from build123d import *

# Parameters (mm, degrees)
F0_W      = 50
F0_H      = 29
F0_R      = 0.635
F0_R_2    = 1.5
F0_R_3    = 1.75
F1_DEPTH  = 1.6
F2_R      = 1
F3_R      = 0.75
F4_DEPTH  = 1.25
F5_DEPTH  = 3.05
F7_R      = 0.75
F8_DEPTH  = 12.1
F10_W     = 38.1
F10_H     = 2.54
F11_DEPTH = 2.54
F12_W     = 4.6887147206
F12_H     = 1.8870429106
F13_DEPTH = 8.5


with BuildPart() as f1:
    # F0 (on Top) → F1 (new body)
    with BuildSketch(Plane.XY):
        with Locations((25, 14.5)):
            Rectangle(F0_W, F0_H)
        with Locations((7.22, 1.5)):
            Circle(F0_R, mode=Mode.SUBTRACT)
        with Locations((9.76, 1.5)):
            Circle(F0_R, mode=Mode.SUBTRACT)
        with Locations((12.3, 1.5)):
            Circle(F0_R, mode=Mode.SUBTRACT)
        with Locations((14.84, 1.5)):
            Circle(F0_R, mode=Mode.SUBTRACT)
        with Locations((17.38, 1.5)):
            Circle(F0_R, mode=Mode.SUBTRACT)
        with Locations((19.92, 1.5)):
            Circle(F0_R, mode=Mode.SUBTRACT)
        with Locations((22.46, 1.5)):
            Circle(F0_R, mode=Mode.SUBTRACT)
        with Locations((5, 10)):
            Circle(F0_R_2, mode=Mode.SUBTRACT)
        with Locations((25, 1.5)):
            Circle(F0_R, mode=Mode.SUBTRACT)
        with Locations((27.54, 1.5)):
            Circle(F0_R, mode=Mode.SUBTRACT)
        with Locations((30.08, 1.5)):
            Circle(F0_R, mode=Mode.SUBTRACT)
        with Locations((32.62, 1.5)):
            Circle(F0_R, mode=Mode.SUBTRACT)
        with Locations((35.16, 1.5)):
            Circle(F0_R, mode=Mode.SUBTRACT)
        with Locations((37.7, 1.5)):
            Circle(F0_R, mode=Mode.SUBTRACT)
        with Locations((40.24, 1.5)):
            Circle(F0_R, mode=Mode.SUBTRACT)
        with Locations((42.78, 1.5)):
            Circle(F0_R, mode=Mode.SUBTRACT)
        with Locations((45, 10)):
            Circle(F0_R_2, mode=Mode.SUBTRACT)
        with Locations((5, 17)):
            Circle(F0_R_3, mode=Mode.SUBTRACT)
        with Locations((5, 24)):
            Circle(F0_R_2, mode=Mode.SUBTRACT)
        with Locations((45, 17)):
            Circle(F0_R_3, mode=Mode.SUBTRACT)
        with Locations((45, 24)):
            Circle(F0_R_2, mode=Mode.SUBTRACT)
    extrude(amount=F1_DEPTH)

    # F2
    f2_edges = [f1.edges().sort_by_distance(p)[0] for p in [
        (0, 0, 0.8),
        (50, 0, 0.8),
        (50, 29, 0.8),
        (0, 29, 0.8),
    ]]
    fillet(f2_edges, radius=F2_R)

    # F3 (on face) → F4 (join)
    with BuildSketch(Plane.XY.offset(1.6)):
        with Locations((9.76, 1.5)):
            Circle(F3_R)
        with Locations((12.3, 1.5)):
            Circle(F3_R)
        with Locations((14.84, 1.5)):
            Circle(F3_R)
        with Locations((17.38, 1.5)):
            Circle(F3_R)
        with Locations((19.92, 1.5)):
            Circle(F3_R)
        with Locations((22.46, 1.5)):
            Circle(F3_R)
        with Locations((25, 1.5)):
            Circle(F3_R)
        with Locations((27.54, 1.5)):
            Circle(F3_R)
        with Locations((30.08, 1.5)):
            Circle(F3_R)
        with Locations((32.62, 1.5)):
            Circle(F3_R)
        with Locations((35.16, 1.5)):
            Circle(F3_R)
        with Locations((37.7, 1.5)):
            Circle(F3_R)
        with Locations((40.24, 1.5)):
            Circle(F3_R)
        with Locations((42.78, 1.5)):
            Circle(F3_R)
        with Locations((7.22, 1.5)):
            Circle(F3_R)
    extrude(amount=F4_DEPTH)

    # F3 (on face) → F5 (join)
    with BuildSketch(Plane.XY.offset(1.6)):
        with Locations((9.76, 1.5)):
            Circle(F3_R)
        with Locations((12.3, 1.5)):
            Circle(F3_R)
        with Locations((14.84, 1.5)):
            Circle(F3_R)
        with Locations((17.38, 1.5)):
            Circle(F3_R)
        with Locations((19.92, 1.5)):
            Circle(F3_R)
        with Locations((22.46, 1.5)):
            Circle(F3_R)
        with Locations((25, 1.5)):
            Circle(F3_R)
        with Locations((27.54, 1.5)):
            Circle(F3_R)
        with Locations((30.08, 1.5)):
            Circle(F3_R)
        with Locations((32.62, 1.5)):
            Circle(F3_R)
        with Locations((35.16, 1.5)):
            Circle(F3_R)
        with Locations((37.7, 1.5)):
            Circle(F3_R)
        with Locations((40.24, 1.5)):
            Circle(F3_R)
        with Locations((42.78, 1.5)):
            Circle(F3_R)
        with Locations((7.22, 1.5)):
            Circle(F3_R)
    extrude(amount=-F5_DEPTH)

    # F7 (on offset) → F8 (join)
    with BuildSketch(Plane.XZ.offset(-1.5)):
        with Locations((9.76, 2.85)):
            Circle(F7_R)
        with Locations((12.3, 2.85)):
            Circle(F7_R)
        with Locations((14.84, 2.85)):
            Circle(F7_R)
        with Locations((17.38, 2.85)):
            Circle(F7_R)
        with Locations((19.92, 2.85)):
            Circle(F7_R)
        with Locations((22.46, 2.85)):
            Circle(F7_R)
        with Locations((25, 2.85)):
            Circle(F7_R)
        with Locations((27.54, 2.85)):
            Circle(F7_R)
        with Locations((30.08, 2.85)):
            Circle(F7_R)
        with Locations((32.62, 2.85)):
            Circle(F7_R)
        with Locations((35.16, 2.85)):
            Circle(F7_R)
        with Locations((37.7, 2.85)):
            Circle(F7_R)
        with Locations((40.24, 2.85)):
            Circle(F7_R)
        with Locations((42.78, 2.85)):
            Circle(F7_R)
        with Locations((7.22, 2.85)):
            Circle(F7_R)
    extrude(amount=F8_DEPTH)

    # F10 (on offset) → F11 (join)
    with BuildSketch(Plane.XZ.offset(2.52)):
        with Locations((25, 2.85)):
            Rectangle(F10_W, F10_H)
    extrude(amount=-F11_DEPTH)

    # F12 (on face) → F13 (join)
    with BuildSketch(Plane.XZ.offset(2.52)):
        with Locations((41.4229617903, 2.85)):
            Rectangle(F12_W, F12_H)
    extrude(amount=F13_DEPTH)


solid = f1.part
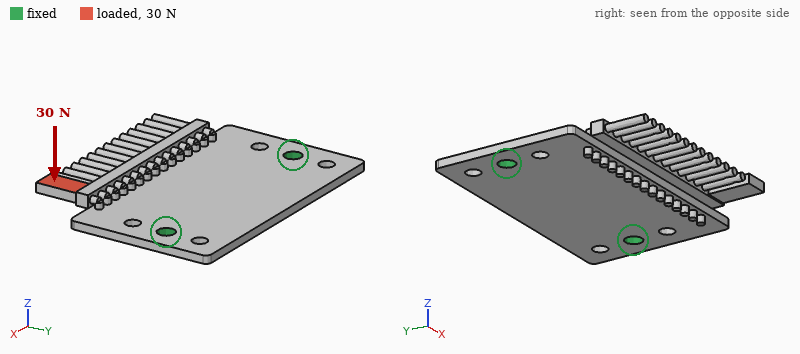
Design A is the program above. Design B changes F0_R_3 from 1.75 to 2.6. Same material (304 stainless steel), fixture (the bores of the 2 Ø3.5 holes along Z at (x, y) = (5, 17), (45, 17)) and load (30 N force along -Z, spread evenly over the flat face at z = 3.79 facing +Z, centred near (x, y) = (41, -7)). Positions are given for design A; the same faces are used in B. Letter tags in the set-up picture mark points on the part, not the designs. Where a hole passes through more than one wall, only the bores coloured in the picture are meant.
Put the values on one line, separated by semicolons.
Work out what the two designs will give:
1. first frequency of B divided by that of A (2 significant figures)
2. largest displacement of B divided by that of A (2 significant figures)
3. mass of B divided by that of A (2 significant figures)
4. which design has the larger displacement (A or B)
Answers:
1.1; 0.91; 0.99; A
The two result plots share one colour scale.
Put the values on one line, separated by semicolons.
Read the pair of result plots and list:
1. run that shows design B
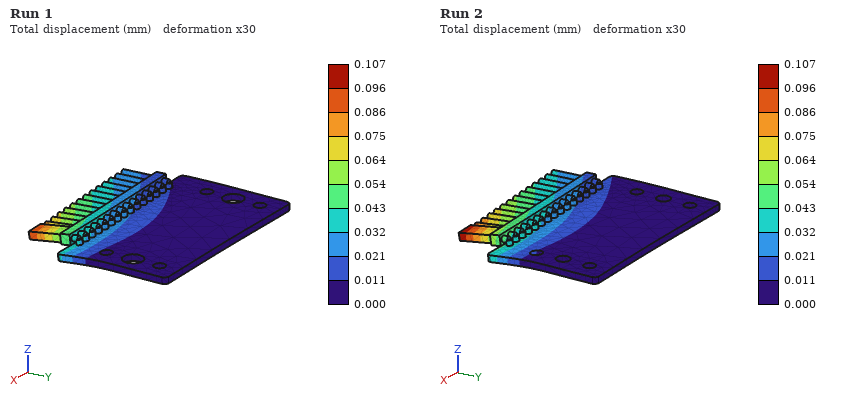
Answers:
Run 1
